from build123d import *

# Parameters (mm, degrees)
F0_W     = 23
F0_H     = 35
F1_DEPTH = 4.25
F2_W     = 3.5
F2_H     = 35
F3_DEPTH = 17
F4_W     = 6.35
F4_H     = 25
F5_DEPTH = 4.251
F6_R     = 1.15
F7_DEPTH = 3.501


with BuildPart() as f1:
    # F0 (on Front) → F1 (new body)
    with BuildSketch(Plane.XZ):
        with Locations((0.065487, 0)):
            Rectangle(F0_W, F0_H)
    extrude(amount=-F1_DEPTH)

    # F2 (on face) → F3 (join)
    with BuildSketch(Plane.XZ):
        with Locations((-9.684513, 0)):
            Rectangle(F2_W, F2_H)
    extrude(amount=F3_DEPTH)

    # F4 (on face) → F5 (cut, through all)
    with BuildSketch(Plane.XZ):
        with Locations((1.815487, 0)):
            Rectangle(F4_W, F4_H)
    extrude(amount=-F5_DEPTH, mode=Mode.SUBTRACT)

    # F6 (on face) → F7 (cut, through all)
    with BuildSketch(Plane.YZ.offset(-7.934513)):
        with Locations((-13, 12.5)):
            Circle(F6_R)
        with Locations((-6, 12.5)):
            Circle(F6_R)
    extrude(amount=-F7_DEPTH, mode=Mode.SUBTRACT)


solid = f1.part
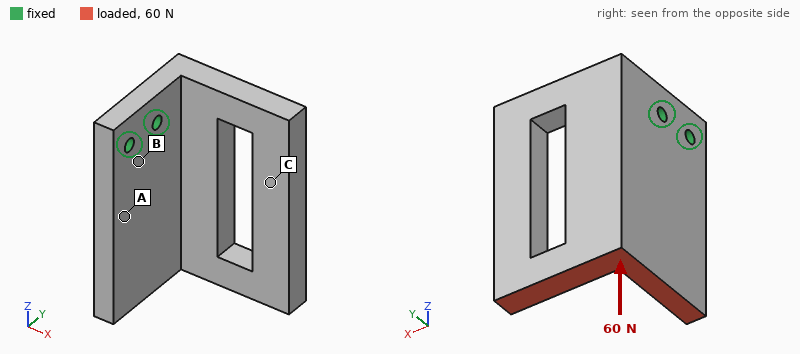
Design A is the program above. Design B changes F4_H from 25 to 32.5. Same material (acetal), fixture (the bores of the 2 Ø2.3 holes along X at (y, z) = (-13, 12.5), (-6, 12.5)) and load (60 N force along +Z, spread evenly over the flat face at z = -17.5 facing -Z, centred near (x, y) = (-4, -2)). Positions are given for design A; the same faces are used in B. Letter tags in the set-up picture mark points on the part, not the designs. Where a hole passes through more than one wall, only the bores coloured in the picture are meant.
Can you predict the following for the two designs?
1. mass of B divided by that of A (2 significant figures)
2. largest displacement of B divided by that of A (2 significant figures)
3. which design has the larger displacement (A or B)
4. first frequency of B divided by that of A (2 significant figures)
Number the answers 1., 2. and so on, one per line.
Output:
1. 0.96
2. 1.3
3. B
4. 0.99
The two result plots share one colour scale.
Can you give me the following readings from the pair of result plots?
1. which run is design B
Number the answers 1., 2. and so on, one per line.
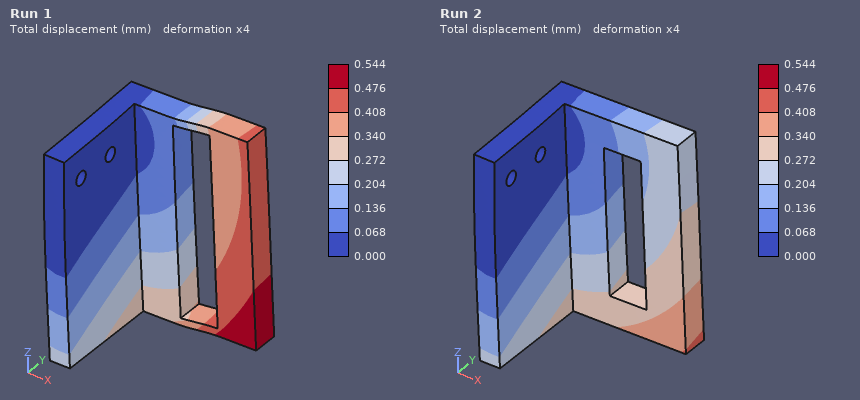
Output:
1. Run 1
